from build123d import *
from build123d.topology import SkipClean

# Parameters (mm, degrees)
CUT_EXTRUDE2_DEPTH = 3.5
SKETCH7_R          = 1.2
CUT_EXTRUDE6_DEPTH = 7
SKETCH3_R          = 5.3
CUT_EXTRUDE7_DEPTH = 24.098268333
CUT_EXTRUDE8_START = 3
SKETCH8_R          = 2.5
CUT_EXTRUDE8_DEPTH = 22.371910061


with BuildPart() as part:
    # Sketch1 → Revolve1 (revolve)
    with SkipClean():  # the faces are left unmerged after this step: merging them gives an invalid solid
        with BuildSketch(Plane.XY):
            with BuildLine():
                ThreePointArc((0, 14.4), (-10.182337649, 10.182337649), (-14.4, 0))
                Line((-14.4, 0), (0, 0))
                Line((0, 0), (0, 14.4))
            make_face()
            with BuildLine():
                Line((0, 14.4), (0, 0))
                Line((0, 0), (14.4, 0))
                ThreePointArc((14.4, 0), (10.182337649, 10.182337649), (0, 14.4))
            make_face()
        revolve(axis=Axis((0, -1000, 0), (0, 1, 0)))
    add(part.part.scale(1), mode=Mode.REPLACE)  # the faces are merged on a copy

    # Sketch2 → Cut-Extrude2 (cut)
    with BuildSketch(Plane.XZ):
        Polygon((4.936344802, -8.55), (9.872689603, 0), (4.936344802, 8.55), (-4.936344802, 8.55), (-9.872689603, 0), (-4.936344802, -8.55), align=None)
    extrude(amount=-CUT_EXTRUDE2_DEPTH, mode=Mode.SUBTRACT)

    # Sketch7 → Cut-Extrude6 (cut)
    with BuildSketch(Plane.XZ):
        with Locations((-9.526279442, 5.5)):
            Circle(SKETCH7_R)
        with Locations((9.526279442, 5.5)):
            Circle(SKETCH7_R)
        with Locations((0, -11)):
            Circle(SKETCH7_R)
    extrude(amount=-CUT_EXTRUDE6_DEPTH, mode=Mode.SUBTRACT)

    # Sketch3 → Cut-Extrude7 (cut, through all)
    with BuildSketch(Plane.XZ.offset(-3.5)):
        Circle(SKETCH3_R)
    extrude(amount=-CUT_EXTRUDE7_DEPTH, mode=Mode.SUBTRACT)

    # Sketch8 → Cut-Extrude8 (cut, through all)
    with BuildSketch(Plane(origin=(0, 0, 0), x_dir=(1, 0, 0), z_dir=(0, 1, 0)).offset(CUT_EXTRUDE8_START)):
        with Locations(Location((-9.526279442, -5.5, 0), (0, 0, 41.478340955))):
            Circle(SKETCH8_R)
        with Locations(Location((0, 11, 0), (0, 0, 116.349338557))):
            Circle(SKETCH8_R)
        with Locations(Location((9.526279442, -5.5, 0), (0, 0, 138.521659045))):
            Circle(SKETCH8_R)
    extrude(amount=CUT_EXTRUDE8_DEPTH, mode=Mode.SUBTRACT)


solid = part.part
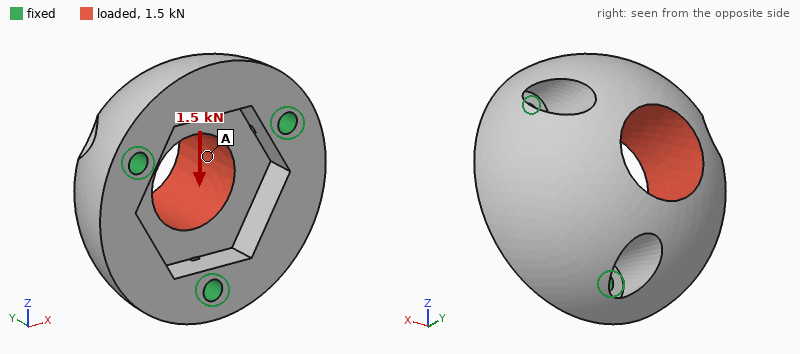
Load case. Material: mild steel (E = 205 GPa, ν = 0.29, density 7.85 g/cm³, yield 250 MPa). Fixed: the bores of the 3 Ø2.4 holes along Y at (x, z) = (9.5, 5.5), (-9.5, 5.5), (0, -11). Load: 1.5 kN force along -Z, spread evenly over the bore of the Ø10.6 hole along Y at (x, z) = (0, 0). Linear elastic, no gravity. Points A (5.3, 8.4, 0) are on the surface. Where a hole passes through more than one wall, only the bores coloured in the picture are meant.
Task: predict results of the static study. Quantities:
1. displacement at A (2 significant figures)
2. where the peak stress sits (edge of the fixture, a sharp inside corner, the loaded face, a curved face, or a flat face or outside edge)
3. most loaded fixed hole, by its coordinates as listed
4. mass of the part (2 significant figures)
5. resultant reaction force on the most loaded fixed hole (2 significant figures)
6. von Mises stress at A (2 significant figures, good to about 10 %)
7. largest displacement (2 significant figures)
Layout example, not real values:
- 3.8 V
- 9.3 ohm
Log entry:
- 2.2 µm
- a flat face or outside edge
- (0, -11)
- 32 g
- 750 N
- 17 MPa
- 3.7 µm
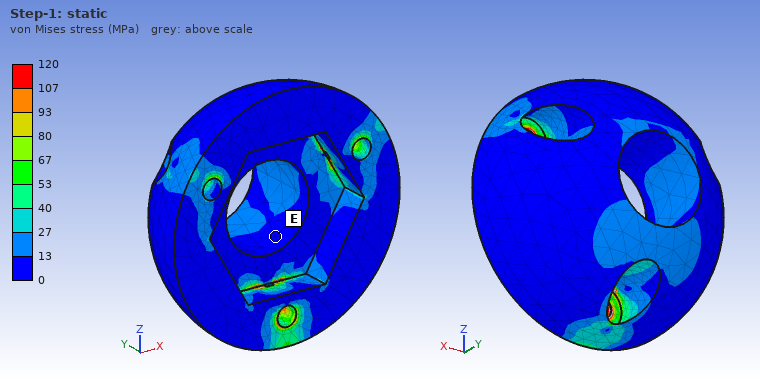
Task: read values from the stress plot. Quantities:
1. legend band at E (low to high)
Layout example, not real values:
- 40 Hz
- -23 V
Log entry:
- 0 to 13 MPa
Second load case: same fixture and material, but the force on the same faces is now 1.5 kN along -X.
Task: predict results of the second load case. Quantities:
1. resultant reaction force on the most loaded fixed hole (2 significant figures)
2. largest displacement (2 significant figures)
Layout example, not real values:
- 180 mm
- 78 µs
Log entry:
- 690 N
- 3.5 µm
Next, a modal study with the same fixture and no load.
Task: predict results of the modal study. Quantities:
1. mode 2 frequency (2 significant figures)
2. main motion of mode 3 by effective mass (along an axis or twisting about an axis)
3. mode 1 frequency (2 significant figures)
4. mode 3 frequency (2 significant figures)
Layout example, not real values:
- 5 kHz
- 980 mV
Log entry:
- 26 kHz
- along Y
- 26 kHz
- 33 kHz
